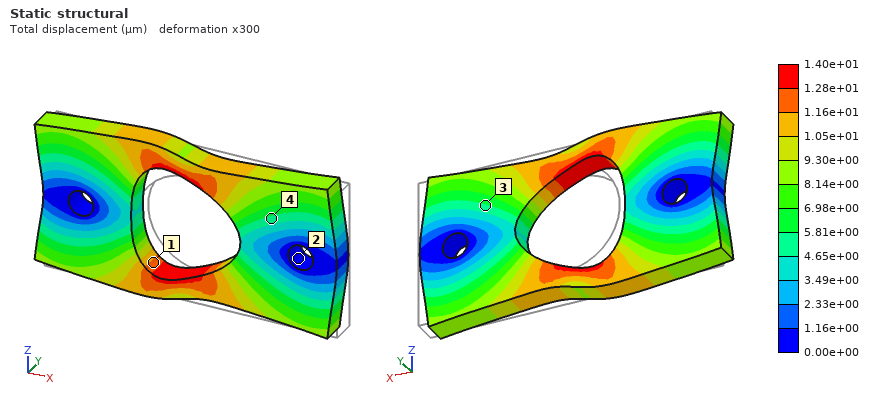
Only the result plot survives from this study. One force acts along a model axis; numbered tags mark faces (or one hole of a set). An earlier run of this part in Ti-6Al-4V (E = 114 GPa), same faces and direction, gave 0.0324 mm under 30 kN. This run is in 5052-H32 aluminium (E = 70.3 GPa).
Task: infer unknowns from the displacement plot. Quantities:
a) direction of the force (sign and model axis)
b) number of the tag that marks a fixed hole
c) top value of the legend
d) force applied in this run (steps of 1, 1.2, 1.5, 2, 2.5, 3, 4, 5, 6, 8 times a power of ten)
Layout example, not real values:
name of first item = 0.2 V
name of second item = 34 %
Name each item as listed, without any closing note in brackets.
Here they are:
direction of the force = -X
number of the tag that marks a fixed hole = 2
top value of the legend = 1.40e+01 µm
force applied in this run = 8 kN
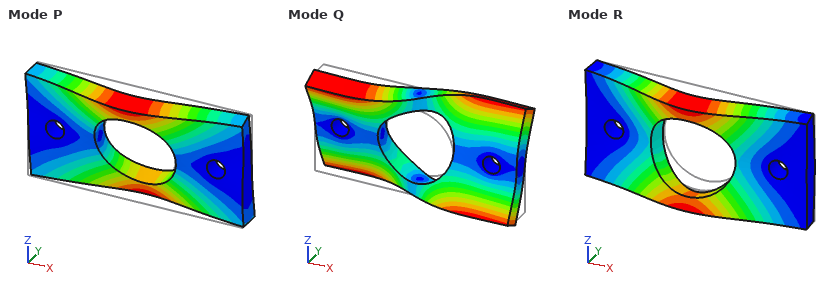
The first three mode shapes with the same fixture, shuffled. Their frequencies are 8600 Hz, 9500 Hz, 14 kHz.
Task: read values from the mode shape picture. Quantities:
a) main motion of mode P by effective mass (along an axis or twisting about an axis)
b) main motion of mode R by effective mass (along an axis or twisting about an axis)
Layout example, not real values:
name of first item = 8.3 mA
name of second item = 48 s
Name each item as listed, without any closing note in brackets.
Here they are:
main motion of mode P by effective mass = twisting about X
main motion of mode R by effective mass = along Y
